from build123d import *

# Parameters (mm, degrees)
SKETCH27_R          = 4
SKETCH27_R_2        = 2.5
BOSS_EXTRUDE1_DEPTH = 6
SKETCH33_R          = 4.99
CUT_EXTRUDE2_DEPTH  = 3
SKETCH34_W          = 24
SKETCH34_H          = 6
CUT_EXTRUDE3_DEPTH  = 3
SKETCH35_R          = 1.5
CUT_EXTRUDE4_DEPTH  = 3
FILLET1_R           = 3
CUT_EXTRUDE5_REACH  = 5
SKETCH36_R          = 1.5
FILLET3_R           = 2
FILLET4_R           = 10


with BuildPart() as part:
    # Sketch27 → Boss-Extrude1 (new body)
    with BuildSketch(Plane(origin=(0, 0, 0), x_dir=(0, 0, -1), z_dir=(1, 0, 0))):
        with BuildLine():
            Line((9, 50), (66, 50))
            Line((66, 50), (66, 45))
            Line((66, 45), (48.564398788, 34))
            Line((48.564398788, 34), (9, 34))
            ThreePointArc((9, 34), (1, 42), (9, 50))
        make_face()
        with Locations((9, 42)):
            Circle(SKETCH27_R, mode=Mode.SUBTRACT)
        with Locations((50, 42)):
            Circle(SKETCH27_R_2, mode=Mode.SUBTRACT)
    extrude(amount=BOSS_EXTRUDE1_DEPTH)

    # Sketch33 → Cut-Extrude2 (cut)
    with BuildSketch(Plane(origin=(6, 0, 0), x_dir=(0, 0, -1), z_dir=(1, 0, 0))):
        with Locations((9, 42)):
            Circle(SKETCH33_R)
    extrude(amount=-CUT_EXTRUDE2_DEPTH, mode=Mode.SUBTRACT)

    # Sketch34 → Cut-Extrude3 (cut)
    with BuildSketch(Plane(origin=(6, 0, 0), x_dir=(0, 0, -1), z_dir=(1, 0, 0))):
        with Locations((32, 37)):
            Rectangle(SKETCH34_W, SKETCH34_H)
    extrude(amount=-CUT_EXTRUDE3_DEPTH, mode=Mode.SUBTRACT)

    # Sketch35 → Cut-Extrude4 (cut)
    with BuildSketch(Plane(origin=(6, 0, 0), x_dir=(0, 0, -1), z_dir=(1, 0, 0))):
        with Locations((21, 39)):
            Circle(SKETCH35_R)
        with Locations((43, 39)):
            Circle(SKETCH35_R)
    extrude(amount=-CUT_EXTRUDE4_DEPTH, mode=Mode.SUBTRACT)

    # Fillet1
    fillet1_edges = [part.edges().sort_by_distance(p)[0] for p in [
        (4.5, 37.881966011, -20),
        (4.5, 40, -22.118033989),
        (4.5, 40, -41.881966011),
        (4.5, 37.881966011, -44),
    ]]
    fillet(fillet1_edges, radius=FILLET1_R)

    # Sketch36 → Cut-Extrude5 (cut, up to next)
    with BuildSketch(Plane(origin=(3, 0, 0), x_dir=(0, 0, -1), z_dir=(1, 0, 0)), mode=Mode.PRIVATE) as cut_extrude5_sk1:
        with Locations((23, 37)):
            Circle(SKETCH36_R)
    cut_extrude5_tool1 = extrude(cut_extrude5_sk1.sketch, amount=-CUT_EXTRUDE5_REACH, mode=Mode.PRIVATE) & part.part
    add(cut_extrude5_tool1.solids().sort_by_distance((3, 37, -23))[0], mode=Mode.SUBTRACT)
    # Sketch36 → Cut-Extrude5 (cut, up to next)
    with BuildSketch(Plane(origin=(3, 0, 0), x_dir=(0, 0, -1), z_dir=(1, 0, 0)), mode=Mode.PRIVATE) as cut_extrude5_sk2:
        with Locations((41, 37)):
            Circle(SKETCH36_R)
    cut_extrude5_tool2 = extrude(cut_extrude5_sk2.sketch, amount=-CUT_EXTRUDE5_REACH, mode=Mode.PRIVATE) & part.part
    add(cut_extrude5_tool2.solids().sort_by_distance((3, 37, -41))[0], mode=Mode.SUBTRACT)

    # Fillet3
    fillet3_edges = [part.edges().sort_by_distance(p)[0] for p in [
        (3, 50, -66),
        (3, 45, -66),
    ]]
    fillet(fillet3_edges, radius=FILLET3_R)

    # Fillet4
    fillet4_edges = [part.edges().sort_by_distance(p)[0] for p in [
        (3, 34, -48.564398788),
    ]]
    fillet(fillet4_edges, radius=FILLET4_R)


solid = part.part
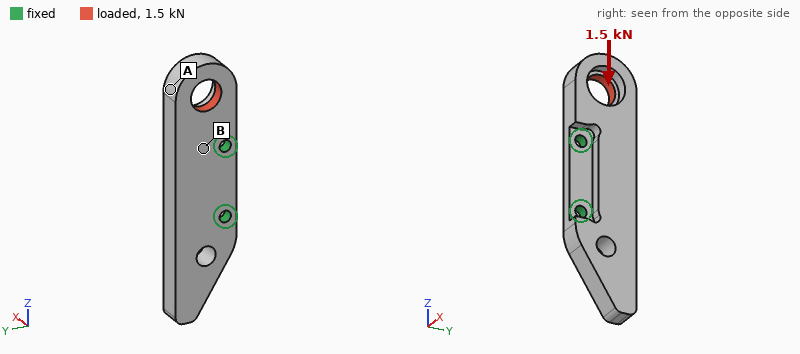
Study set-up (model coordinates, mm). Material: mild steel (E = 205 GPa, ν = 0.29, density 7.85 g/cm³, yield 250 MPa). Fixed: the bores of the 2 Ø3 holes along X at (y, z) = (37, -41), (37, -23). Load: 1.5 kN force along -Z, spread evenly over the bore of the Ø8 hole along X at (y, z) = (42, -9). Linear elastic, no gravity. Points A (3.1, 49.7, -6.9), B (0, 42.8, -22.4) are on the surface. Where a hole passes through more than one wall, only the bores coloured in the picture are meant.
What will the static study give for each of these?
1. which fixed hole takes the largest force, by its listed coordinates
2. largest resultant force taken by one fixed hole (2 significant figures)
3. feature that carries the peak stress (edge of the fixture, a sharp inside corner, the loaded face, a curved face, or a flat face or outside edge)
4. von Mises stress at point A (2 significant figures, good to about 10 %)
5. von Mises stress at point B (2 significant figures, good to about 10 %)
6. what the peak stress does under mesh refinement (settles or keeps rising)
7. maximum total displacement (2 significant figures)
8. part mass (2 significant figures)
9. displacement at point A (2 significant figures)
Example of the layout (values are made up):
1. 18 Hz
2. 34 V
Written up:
1. (37, -23)
2. 1.2 kN
3. edge of the fixture
4. 12 MPa
5. 30 MPa
6. keeps rising
7. 13 µm
8. 35 g
9. 8.8 µm
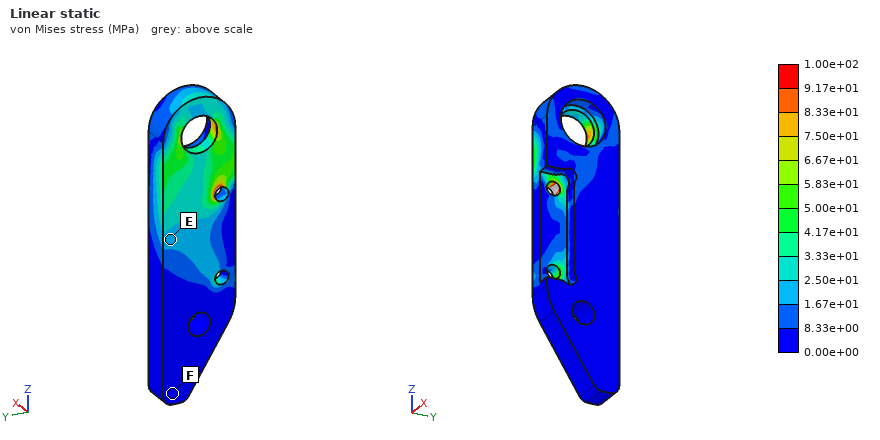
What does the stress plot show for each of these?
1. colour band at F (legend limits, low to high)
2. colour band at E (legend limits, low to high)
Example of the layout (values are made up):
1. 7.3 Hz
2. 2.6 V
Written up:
1. 0.00e+00 to 8.33e+00 MPa
2. 1.67e+01 to 2.50e+01 MPa
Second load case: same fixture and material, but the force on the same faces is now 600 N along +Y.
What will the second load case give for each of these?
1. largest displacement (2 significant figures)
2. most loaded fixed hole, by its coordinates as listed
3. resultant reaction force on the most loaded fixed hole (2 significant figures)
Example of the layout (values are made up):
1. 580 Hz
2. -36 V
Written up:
1. 14 µm
2. (37, -23)
3. 1.0 kN
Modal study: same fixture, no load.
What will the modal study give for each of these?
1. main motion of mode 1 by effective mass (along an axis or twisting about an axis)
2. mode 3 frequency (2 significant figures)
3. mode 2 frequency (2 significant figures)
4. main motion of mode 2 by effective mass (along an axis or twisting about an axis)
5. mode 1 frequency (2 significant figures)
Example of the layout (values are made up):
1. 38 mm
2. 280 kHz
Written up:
1. along X
2. 10 kHz
3. 7100 Hz
4. along X
5. 5600 Hz
